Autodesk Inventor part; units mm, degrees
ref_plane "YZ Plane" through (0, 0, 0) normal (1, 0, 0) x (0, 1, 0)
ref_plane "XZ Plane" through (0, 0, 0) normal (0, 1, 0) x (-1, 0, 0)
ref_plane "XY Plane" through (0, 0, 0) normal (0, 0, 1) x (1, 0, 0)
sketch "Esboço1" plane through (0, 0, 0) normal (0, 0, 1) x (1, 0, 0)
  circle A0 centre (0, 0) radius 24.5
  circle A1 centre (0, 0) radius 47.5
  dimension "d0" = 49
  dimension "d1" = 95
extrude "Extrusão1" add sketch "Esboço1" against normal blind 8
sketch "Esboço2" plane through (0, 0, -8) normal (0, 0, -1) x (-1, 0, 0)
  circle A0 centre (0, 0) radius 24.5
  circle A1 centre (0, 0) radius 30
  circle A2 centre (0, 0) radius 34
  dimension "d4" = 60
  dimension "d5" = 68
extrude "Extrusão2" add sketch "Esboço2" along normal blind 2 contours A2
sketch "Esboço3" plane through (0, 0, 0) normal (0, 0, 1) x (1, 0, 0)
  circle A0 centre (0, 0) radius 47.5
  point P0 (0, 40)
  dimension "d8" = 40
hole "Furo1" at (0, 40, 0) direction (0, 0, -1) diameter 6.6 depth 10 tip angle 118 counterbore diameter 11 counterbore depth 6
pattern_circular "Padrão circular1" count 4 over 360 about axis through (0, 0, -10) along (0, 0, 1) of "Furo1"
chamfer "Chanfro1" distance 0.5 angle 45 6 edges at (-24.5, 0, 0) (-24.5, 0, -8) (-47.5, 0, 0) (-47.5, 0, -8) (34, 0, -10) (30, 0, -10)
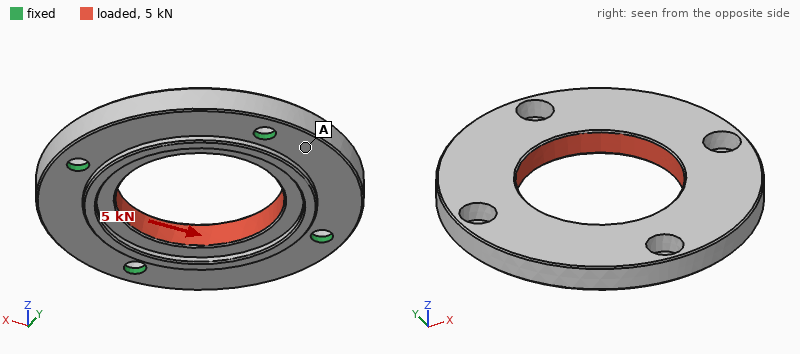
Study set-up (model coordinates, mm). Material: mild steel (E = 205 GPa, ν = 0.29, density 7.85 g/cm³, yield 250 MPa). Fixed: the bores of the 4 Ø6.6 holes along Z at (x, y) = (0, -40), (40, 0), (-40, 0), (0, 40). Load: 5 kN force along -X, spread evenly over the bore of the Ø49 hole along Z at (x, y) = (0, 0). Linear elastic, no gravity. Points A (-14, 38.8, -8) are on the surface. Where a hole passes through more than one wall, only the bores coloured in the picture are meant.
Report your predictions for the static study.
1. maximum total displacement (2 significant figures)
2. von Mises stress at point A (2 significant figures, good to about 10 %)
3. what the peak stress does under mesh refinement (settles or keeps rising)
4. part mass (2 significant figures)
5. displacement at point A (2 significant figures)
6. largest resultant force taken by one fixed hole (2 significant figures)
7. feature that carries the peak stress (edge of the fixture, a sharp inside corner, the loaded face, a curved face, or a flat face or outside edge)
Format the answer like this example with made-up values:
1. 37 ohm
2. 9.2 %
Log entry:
1. 2.9 µm
2. 9.6 MPa
3. keeps rising
4. 320 g
5. 1.5 µm
6. 1.3 kN
7. edge of the fixture
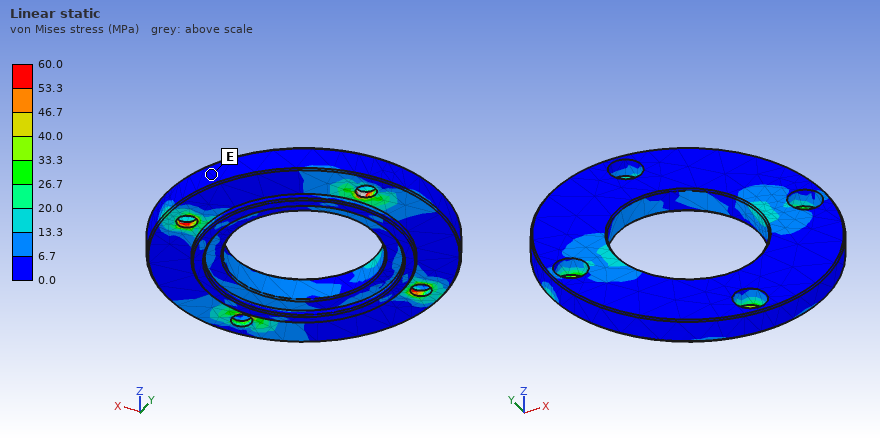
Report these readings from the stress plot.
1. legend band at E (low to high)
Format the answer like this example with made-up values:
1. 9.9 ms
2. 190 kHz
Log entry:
1. 0.0 to 6.7 MPa
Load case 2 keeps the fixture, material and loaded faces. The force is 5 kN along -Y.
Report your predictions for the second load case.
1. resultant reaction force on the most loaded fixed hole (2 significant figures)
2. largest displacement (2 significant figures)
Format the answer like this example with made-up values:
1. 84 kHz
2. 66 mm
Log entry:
1. 1.3 kN
2. 2.9 µm
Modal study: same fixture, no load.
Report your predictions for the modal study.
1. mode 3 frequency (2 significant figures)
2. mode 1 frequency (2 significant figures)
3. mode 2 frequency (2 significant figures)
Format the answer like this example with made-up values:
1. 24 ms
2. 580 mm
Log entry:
1. 7300 Hz
2. 5700 Hz
3. 7300 Hz
